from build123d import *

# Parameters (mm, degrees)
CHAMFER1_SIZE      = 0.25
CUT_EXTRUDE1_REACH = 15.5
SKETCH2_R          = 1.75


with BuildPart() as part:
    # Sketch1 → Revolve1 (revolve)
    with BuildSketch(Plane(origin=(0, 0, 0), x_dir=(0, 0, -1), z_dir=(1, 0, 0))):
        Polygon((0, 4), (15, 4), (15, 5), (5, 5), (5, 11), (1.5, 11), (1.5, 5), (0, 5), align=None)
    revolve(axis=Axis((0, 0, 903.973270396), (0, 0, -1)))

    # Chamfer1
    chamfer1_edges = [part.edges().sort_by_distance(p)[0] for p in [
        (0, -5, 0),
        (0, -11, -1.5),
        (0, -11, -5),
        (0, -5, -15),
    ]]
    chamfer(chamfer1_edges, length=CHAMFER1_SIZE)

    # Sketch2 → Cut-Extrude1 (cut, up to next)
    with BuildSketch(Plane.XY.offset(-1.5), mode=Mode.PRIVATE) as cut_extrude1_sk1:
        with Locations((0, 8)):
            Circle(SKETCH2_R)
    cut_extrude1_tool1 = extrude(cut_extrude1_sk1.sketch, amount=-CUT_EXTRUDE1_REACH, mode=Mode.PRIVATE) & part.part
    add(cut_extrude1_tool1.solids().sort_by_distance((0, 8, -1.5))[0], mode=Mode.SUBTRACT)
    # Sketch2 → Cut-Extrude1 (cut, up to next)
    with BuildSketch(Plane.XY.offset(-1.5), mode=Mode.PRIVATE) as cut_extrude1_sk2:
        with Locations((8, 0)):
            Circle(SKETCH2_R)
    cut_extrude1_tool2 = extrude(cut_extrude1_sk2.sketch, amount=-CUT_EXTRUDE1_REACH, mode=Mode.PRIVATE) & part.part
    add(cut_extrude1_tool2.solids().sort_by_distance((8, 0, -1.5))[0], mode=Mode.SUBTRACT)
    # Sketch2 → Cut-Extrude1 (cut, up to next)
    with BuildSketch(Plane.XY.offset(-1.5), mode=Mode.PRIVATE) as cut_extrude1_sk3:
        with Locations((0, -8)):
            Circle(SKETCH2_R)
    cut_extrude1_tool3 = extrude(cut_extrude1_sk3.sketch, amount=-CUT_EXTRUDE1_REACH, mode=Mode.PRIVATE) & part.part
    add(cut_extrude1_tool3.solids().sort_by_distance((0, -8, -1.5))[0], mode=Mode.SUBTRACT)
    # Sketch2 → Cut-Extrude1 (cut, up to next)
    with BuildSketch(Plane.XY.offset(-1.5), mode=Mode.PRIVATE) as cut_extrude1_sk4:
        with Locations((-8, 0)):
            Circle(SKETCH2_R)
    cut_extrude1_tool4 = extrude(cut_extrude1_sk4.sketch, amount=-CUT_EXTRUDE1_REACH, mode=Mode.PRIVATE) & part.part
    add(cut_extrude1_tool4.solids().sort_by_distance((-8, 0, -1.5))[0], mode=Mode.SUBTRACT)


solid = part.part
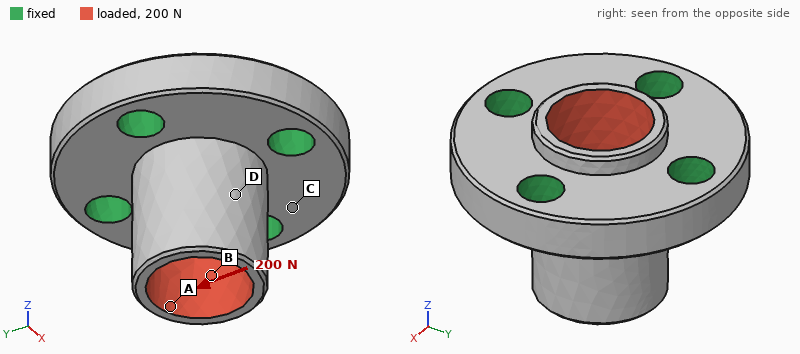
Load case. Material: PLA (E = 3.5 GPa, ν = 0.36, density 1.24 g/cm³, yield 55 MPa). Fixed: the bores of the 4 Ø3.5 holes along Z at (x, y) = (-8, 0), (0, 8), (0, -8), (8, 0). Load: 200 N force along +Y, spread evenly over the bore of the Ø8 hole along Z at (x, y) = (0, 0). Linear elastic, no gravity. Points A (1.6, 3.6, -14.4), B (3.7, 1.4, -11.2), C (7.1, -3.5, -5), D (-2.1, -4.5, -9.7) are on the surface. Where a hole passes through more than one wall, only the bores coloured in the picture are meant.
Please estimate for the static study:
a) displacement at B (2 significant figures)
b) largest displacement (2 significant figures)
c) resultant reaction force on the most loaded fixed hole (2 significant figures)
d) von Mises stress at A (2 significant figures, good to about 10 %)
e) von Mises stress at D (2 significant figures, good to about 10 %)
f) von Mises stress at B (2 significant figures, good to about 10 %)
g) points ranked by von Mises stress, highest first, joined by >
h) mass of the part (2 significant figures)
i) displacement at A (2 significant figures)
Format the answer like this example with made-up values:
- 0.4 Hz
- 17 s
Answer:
- 51 µm
- 75 µm
- 84 N
- 2.8 MPa
- 4.8 MPa
- 6.4 MPa
- B > D > A > C
- 1.7 g
- 71 µm
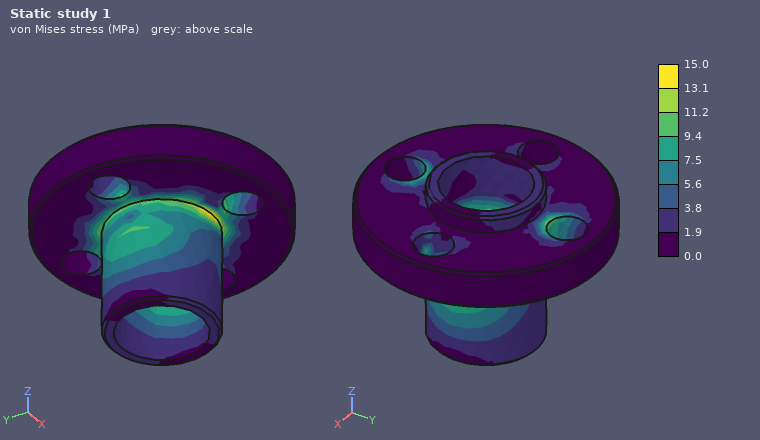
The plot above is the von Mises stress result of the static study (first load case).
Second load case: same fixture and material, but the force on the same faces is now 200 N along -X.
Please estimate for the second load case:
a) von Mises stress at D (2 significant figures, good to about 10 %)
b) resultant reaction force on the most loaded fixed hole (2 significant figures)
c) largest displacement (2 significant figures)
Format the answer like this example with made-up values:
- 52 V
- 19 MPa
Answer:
- 7.3 MPa
- 84 N
- 75 µm
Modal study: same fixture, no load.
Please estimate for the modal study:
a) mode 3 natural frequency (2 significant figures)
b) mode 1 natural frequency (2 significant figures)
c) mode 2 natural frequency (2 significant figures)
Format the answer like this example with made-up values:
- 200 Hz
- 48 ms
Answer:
- 13 kHz
- 13 kHz
- 13 kHz
